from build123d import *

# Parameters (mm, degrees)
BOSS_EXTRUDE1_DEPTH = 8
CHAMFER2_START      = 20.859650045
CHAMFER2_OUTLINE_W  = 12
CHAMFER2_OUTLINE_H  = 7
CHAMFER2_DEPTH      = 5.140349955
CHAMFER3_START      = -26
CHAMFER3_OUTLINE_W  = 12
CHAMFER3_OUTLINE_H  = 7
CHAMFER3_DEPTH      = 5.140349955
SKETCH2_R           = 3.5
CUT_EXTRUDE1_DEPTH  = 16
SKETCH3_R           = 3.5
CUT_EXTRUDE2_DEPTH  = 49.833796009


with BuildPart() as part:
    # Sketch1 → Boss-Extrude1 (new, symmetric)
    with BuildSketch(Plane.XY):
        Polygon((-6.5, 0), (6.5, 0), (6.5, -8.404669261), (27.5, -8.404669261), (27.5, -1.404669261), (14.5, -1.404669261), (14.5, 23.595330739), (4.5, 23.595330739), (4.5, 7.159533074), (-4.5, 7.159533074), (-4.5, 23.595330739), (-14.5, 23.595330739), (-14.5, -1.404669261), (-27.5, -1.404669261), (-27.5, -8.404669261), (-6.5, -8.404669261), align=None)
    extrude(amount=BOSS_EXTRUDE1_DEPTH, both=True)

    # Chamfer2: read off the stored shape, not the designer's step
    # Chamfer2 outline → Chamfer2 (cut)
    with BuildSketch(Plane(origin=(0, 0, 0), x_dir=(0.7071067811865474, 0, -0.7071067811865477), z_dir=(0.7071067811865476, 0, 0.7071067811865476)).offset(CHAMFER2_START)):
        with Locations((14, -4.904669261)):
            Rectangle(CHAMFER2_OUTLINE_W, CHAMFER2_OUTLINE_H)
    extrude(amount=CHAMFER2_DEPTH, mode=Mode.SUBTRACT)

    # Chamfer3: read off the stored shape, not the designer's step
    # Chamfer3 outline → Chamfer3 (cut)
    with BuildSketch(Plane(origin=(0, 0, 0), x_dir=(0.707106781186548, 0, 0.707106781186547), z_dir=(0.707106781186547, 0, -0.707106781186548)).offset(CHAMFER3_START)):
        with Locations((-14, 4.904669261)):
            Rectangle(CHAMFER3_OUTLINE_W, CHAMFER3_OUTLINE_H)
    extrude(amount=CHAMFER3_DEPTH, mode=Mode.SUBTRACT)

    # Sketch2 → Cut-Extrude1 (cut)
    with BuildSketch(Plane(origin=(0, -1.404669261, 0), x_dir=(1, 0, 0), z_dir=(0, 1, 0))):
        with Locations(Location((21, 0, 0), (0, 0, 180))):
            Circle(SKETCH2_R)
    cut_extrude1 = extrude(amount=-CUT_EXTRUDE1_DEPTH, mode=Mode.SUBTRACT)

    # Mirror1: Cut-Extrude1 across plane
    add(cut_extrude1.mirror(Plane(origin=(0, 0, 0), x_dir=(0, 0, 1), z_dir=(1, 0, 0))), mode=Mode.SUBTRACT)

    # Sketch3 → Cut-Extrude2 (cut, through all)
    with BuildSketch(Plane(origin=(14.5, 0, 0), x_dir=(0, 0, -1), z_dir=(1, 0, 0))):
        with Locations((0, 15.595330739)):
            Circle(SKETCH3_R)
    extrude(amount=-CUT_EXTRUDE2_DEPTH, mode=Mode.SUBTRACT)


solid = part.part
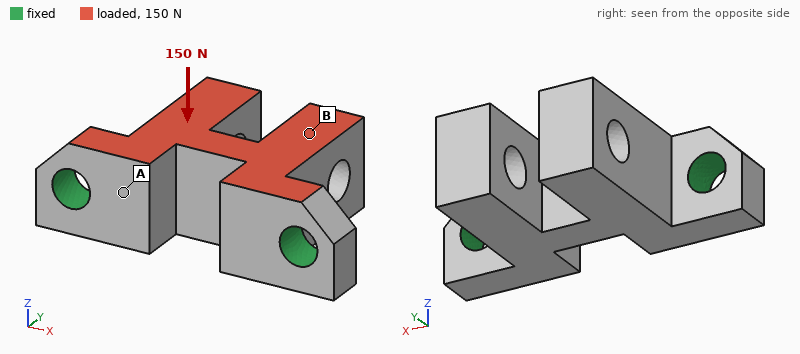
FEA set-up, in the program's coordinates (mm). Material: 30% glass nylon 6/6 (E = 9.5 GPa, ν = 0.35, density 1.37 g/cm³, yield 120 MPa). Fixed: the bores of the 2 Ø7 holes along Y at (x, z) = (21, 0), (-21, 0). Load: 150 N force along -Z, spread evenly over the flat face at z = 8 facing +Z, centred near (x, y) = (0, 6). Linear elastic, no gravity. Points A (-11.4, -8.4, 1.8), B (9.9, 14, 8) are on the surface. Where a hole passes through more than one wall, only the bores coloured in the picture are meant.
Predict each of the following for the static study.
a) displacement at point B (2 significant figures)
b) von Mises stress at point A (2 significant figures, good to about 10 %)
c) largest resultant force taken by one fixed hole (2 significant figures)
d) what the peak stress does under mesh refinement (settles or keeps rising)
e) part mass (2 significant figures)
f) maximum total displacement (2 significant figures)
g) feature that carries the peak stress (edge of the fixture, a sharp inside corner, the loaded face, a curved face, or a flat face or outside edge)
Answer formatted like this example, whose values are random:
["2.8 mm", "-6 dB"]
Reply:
["26 µm", "1.7 MPa", "75 N", "keeps rising", "17 g", "37 µm", "edge of the fixture"]
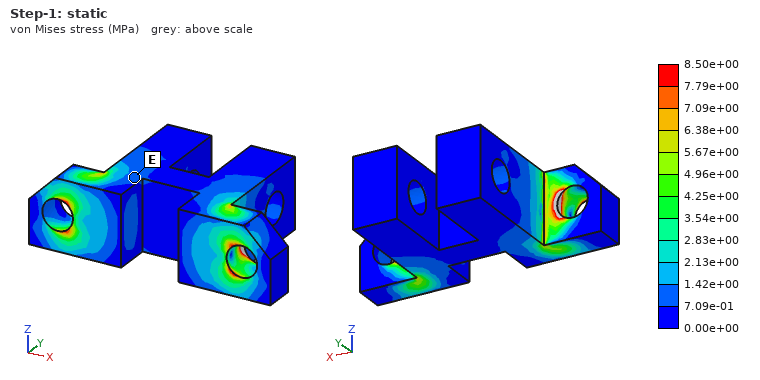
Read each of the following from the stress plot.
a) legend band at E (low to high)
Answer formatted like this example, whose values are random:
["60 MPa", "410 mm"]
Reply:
["7.09e-01 to 1.42e+00 MPa"]
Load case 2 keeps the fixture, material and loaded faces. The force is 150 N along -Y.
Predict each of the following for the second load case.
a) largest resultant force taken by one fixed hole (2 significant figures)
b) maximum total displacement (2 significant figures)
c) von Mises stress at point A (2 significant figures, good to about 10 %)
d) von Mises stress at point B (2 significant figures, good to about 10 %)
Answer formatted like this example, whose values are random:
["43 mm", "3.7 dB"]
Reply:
["85 N", "23 µm", "1.6 MPa", "0.66 MPa"]
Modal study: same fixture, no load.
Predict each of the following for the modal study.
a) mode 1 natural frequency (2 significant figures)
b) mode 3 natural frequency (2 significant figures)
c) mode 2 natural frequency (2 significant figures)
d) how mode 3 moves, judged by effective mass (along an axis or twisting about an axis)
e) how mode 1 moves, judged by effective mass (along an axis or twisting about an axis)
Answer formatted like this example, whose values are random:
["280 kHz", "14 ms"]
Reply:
["3200 Hz", "6600 Hz", "5600 Hz", "along X", "along Z"]
